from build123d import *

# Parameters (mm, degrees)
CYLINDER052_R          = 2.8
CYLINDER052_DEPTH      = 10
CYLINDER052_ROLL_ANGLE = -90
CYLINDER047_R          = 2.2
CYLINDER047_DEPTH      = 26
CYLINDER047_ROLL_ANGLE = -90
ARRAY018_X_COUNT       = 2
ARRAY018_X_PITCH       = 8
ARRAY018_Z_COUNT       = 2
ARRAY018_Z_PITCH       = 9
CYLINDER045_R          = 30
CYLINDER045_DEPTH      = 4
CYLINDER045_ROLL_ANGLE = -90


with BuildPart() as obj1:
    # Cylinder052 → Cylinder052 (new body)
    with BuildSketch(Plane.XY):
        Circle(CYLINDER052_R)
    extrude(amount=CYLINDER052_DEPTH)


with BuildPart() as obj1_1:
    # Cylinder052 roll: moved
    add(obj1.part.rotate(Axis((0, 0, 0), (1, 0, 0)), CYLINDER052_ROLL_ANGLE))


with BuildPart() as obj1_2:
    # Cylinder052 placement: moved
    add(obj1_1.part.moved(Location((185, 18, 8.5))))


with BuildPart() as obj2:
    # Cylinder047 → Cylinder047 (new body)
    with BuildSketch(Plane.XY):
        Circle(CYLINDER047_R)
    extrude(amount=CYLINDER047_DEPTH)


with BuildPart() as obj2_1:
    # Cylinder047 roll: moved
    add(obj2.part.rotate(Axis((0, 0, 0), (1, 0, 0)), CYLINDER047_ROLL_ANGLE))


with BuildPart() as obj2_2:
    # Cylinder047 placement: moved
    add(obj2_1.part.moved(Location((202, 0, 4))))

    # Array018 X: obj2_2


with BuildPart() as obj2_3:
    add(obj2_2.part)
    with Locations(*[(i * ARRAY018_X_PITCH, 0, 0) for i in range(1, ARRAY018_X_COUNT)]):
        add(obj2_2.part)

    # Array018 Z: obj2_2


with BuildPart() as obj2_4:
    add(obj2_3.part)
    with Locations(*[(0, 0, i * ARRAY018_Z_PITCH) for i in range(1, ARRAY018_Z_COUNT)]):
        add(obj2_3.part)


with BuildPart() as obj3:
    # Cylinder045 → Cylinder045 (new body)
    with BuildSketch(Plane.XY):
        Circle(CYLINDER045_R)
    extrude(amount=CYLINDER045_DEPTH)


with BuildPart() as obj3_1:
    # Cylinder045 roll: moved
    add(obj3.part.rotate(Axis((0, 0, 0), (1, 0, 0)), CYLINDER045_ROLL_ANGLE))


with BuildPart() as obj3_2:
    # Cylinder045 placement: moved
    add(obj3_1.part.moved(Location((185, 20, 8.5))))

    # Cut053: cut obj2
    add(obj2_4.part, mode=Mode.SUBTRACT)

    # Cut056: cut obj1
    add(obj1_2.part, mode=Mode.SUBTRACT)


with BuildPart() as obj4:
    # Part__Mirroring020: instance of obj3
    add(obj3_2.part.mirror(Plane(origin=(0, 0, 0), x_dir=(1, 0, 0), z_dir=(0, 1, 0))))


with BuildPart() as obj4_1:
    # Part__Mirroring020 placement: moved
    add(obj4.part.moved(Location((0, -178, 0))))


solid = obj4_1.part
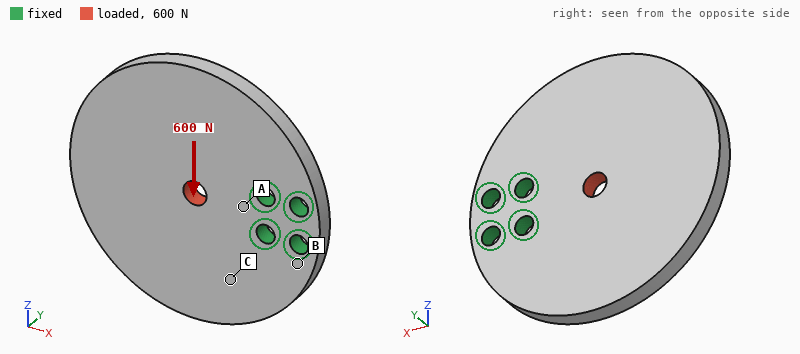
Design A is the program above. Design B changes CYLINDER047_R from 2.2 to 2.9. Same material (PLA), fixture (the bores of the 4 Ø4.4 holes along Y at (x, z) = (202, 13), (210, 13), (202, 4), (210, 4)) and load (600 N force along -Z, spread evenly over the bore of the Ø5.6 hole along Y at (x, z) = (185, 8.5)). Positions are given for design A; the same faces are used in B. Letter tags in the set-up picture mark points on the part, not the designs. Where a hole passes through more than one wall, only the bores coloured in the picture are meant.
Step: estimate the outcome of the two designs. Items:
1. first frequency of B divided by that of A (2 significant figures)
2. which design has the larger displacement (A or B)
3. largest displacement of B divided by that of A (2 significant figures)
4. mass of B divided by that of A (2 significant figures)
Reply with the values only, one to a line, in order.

1.0
A
0.84
0.98
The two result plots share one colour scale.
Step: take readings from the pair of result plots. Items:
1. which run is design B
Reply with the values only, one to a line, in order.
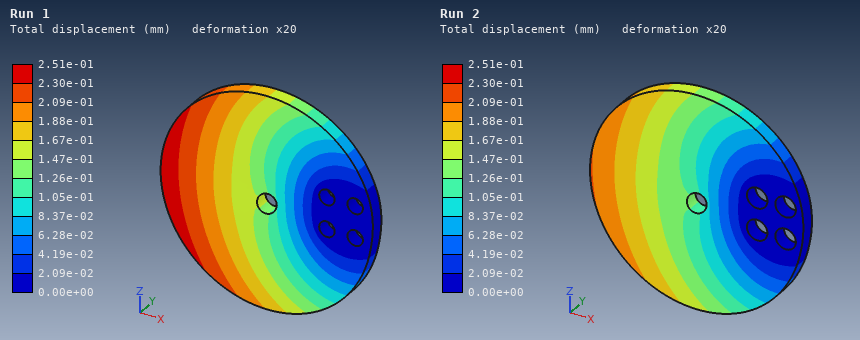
Run 2
